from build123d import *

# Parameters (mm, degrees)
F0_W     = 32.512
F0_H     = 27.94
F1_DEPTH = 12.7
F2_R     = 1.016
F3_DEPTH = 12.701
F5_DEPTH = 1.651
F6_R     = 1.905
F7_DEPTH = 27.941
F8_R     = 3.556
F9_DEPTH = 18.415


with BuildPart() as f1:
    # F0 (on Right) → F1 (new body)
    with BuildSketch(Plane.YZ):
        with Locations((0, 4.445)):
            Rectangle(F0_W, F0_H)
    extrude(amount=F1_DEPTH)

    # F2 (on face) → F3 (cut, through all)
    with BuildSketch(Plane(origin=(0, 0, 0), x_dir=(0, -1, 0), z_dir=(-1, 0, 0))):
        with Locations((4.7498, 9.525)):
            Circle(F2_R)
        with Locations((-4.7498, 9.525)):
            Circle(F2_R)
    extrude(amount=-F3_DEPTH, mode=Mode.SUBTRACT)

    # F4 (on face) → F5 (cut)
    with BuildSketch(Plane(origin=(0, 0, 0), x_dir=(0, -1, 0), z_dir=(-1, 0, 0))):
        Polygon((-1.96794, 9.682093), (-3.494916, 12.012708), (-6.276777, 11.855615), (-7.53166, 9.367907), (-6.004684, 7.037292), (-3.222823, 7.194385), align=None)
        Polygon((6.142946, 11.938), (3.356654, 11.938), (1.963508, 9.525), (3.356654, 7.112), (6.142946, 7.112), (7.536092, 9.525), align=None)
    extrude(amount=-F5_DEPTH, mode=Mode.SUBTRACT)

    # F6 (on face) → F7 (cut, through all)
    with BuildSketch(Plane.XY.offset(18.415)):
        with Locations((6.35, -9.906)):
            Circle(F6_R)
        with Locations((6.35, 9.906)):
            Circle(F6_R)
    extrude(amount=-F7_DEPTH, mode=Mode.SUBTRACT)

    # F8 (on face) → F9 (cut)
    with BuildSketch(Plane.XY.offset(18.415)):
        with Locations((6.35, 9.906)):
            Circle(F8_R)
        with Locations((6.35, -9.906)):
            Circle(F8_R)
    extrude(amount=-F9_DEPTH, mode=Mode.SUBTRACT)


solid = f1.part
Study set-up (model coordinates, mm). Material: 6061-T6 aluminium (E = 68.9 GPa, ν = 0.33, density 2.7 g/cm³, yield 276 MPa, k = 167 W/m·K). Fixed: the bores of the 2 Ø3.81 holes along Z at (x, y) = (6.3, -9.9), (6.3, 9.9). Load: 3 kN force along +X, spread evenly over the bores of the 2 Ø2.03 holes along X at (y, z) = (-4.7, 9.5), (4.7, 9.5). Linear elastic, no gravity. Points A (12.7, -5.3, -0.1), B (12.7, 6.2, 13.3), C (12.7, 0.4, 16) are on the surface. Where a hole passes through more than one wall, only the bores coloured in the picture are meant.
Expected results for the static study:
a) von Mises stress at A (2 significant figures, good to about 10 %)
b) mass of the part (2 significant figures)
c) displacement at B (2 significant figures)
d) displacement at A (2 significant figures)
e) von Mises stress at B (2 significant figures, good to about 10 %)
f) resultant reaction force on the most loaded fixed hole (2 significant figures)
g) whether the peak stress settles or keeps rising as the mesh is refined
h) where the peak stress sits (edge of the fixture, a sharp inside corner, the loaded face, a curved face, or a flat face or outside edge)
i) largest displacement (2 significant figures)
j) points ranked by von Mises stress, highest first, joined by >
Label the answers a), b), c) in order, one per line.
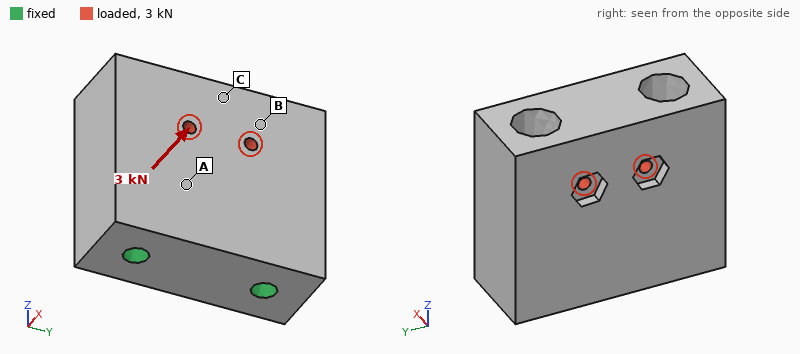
a) 43 MPa
b) 26 g
c) 36 µm
d) 12 µm
e) 25 MPa
f) 1.5 kN
g) keeps rising
h) edge of the fixture
i) 45 µm
j) A > B > C
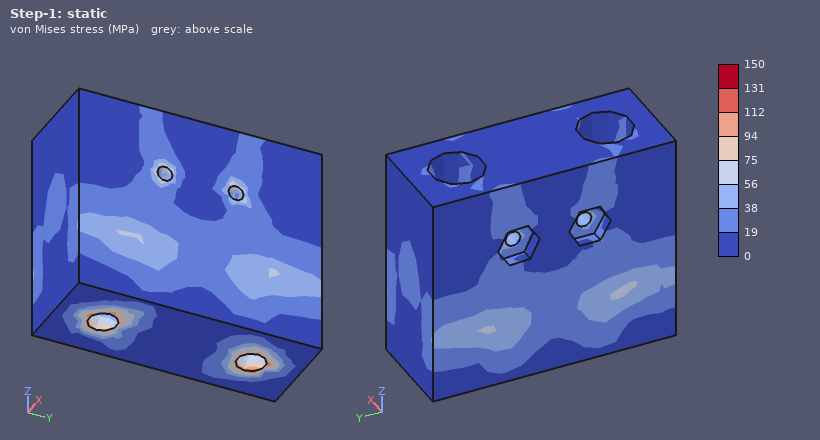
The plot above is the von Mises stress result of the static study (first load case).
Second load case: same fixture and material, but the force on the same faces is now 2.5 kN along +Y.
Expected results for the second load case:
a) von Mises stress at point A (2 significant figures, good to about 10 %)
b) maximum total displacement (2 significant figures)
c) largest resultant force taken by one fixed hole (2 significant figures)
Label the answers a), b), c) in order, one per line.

a) 13 MPa
b) 9.9 µm
c) 1.9 kN
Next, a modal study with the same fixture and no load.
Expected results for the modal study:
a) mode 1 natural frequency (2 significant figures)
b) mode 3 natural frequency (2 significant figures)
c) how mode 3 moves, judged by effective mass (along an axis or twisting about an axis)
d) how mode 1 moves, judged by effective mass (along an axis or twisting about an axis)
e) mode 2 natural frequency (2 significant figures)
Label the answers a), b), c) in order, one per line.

a) 13 kHz
b) 24 kHz
c) twisting about Z
d) along X
e) 23 kHz
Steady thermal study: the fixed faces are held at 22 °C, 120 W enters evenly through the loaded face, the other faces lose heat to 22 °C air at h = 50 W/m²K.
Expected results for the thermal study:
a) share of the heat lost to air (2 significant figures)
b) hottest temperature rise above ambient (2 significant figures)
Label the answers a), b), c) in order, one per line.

a) 3.4 %
b) 44 K
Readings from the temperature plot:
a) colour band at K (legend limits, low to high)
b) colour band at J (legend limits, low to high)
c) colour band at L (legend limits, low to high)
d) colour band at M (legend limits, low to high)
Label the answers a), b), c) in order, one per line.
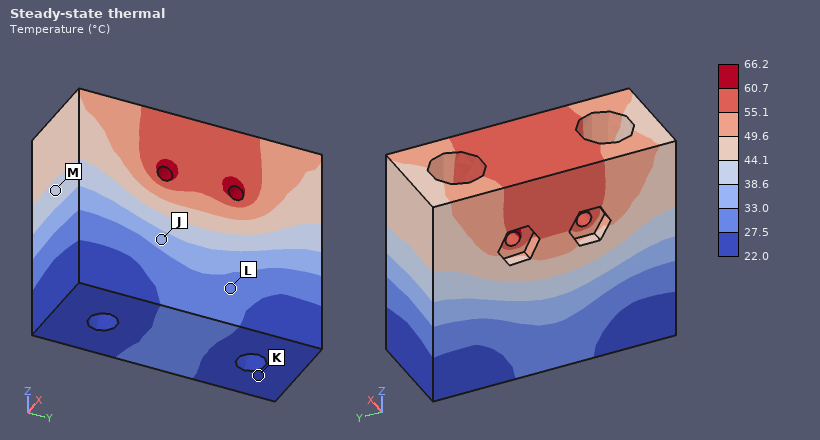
a) 22.0 to 27.5 °C
b) 33.0 to 38.6 °C
c) 27.5 to 33.0 °C
d) 38.6 to 44.1 °C
